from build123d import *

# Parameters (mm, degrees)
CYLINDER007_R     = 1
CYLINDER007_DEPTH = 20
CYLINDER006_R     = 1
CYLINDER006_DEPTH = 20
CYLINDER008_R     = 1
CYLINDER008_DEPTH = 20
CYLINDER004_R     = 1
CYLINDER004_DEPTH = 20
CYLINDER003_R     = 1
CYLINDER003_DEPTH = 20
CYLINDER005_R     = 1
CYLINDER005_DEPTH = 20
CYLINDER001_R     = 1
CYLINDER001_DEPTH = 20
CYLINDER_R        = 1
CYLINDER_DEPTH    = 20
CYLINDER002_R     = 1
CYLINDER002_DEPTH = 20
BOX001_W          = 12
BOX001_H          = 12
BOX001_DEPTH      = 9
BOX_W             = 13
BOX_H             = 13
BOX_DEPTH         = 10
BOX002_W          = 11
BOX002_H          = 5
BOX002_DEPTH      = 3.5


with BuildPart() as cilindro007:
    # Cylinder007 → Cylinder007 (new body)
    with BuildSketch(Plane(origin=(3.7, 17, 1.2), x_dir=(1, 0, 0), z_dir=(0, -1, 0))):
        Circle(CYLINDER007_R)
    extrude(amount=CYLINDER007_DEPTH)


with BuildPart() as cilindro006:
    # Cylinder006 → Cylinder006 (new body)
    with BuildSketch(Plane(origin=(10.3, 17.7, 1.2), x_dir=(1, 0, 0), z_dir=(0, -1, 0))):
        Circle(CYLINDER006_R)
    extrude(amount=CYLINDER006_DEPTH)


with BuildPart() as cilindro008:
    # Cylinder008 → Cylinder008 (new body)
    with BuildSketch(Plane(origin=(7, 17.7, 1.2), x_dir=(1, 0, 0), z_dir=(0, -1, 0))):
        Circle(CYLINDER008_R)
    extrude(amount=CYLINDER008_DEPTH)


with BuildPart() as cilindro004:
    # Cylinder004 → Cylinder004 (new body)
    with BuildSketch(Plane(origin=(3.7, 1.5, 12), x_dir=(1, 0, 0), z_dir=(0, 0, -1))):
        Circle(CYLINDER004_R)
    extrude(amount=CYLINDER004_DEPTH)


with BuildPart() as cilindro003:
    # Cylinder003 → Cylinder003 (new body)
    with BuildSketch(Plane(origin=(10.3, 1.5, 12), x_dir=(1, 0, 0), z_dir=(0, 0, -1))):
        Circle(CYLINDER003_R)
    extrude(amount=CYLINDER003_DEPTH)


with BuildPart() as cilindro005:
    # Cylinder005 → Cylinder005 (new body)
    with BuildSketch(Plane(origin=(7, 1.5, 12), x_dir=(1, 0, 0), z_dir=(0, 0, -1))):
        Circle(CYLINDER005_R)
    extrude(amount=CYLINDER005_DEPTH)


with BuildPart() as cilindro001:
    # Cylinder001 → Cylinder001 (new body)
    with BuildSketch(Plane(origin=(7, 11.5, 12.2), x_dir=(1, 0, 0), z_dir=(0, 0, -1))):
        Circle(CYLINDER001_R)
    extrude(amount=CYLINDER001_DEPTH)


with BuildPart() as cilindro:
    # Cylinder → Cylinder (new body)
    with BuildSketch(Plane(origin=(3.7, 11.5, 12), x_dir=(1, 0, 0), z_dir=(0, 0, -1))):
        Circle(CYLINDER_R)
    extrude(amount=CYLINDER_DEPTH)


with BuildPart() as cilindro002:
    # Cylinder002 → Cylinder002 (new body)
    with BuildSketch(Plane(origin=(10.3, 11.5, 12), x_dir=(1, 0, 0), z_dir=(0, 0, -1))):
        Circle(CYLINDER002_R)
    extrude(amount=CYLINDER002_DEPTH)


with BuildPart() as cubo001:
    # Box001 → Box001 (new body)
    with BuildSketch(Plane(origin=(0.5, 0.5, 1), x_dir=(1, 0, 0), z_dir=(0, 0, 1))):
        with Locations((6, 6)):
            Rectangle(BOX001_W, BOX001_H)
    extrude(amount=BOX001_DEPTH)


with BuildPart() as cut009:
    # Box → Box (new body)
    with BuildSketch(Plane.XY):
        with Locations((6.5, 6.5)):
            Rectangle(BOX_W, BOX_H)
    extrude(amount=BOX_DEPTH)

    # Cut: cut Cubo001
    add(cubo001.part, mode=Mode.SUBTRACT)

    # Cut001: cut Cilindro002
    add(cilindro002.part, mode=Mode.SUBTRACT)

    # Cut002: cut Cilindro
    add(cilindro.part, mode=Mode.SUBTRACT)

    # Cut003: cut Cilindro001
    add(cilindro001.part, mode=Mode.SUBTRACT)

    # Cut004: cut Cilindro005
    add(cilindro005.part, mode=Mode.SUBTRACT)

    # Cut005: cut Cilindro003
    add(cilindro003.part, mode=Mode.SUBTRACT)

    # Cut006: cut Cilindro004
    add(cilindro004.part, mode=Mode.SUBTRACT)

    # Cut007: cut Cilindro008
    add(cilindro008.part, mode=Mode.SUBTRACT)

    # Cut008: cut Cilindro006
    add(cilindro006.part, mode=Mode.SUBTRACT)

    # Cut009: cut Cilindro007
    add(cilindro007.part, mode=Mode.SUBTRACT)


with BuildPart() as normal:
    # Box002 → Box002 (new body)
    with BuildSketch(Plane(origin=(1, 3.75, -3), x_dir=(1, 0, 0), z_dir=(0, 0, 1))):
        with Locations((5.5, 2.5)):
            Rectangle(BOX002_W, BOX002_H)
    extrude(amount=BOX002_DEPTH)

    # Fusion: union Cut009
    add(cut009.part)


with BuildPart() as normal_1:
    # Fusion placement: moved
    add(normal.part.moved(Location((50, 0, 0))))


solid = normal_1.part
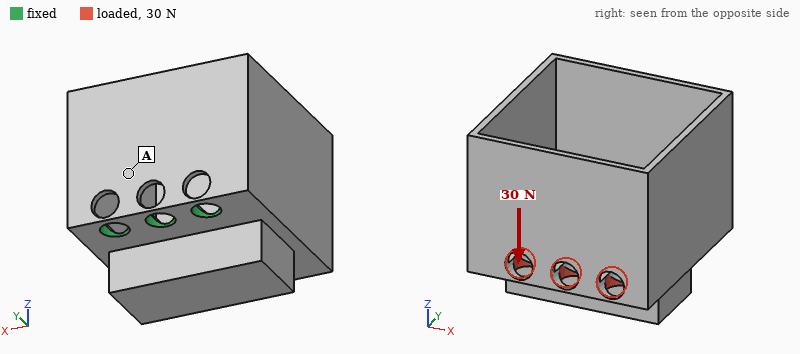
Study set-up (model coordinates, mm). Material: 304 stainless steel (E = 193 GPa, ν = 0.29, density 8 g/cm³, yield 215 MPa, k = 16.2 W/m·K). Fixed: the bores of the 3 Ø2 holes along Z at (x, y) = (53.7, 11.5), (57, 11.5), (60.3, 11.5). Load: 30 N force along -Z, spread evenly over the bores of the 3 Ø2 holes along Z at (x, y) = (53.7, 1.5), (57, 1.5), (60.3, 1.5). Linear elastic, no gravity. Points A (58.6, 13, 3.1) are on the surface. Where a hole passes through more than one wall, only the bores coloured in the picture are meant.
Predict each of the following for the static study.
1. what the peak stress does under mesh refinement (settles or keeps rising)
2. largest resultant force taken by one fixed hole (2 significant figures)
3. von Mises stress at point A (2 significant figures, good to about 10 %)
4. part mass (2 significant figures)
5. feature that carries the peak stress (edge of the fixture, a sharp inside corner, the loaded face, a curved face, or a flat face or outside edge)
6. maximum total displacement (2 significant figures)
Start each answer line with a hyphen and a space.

- keeps rising
- 18 N
- 16 MPa
- 4.0 g
- edge of the fixture
- 24 µm
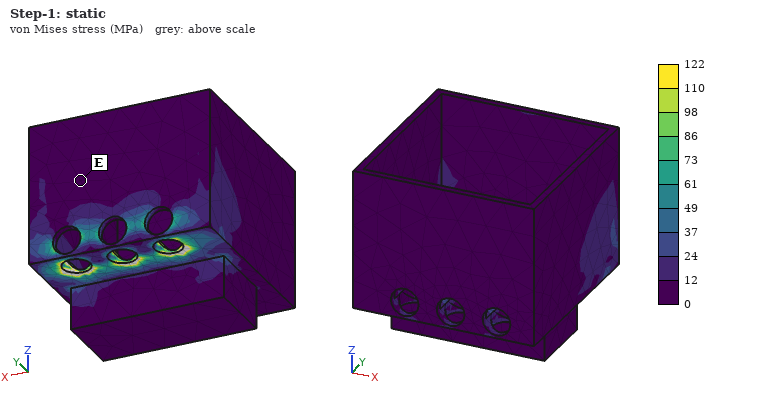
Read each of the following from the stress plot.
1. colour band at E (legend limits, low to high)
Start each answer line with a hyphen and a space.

- 0 to 12 MPa
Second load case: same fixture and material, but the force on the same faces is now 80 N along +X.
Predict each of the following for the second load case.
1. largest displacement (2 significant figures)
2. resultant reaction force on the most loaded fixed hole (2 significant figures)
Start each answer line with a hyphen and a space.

- 6.1 µm
- 97 N
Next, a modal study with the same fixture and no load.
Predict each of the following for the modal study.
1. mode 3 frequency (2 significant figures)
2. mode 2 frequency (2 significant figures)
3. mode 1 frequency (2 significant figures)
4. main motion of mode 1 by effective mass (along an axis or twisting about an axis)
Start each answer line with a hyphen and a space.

- 11 kHz
- 8200 Hz
- 4600 Hz
- along Z
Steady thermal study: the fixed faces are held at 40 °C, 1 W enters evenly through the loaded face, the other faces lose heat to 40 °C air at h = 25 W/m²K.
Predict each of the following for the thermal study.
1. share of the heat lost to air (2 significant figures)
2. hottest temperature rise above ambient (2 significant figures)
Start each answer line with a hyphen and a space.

- 39 %
- 38 K
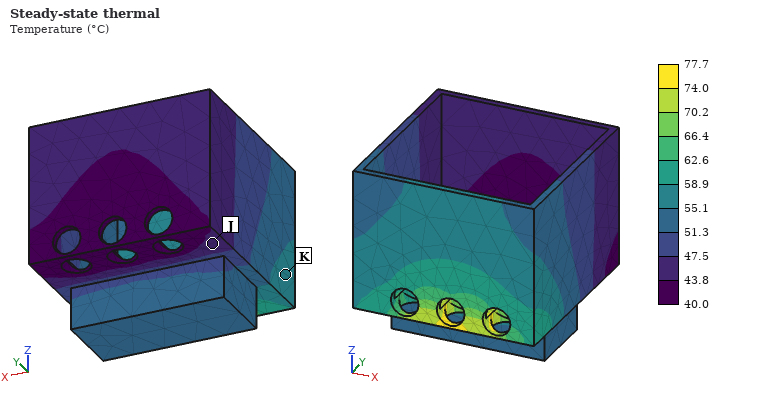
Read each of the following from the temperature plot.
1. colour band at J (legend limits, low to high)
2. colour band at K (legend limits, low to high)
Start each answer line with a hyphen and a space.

- 43.8 to 47.5 °C
- 55.1 to 58.9 °C
